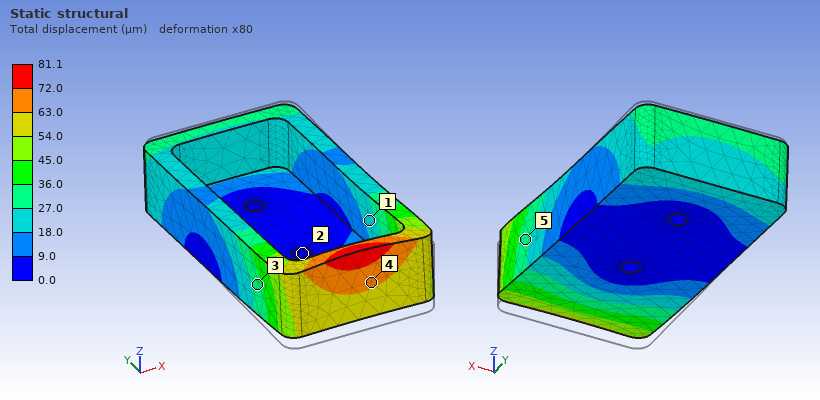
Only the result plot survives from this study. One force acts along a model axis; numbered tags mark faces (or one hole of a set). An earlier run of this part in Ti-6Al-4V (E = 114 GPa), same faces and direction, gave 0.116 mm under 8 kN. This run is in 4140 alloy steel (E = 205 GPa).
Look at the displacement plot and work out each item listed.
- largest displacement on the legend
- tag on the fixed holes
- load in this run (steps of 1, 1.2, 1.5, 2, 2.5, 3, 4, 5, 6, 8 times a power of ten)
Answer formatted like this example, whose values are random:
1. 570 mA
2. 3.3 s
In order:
1. 81.1 µm
2. 2
3. 10 kN
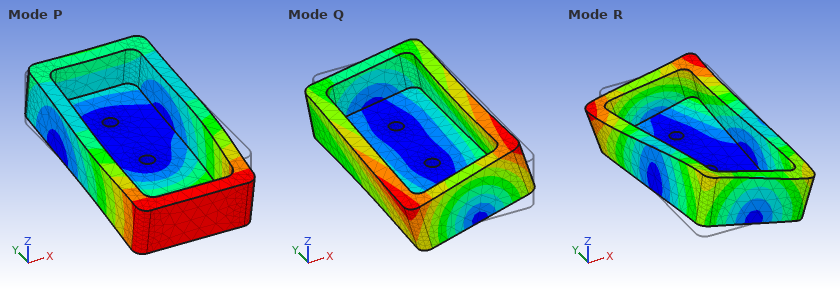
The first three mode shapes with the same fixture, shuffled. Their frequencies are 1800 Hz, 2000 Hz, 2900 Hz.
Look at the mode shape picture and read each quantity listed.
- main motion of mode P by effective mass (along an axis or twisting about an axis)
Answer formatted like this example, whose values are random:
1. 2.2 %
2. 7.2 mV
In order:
1. along Z
